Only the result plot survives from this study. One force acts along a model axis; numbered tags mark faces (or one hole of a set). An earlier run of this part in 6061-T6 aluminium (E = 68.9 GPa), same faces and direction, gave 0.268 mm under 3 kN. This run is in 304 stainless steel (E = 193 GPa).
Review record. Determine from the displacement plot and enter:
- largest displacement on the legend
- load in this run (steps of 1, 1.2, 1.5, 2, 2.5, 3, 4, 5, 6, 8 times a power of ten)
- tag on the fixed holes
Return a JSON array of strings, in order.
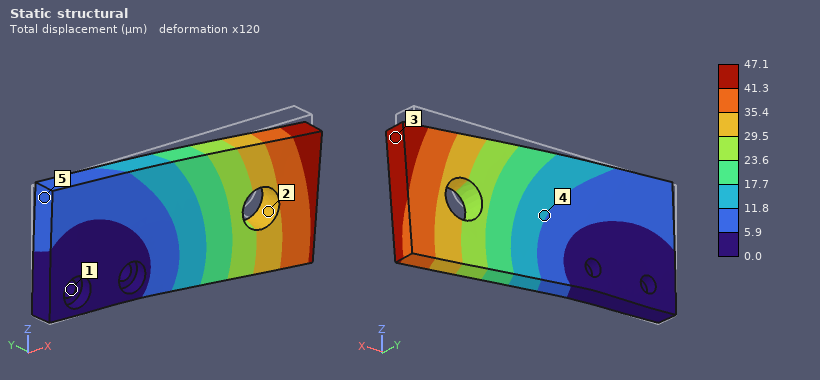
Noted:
["47.1 µm", "1.5 kN", "1"]
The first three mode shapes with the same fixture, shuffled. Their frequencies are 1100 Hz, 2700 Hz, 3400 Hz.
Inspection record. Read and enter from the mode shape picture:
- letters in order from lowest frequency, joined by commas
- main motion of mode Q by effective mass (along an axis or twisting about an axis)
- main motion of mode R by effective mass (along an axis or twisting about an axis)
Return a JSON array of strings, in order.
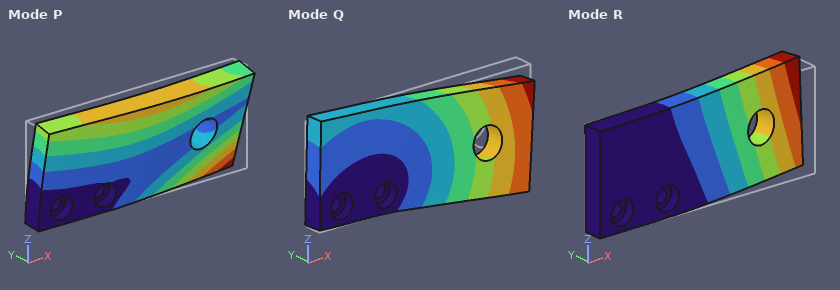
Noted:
["R, P, Q", "along Z", "along Y"]
